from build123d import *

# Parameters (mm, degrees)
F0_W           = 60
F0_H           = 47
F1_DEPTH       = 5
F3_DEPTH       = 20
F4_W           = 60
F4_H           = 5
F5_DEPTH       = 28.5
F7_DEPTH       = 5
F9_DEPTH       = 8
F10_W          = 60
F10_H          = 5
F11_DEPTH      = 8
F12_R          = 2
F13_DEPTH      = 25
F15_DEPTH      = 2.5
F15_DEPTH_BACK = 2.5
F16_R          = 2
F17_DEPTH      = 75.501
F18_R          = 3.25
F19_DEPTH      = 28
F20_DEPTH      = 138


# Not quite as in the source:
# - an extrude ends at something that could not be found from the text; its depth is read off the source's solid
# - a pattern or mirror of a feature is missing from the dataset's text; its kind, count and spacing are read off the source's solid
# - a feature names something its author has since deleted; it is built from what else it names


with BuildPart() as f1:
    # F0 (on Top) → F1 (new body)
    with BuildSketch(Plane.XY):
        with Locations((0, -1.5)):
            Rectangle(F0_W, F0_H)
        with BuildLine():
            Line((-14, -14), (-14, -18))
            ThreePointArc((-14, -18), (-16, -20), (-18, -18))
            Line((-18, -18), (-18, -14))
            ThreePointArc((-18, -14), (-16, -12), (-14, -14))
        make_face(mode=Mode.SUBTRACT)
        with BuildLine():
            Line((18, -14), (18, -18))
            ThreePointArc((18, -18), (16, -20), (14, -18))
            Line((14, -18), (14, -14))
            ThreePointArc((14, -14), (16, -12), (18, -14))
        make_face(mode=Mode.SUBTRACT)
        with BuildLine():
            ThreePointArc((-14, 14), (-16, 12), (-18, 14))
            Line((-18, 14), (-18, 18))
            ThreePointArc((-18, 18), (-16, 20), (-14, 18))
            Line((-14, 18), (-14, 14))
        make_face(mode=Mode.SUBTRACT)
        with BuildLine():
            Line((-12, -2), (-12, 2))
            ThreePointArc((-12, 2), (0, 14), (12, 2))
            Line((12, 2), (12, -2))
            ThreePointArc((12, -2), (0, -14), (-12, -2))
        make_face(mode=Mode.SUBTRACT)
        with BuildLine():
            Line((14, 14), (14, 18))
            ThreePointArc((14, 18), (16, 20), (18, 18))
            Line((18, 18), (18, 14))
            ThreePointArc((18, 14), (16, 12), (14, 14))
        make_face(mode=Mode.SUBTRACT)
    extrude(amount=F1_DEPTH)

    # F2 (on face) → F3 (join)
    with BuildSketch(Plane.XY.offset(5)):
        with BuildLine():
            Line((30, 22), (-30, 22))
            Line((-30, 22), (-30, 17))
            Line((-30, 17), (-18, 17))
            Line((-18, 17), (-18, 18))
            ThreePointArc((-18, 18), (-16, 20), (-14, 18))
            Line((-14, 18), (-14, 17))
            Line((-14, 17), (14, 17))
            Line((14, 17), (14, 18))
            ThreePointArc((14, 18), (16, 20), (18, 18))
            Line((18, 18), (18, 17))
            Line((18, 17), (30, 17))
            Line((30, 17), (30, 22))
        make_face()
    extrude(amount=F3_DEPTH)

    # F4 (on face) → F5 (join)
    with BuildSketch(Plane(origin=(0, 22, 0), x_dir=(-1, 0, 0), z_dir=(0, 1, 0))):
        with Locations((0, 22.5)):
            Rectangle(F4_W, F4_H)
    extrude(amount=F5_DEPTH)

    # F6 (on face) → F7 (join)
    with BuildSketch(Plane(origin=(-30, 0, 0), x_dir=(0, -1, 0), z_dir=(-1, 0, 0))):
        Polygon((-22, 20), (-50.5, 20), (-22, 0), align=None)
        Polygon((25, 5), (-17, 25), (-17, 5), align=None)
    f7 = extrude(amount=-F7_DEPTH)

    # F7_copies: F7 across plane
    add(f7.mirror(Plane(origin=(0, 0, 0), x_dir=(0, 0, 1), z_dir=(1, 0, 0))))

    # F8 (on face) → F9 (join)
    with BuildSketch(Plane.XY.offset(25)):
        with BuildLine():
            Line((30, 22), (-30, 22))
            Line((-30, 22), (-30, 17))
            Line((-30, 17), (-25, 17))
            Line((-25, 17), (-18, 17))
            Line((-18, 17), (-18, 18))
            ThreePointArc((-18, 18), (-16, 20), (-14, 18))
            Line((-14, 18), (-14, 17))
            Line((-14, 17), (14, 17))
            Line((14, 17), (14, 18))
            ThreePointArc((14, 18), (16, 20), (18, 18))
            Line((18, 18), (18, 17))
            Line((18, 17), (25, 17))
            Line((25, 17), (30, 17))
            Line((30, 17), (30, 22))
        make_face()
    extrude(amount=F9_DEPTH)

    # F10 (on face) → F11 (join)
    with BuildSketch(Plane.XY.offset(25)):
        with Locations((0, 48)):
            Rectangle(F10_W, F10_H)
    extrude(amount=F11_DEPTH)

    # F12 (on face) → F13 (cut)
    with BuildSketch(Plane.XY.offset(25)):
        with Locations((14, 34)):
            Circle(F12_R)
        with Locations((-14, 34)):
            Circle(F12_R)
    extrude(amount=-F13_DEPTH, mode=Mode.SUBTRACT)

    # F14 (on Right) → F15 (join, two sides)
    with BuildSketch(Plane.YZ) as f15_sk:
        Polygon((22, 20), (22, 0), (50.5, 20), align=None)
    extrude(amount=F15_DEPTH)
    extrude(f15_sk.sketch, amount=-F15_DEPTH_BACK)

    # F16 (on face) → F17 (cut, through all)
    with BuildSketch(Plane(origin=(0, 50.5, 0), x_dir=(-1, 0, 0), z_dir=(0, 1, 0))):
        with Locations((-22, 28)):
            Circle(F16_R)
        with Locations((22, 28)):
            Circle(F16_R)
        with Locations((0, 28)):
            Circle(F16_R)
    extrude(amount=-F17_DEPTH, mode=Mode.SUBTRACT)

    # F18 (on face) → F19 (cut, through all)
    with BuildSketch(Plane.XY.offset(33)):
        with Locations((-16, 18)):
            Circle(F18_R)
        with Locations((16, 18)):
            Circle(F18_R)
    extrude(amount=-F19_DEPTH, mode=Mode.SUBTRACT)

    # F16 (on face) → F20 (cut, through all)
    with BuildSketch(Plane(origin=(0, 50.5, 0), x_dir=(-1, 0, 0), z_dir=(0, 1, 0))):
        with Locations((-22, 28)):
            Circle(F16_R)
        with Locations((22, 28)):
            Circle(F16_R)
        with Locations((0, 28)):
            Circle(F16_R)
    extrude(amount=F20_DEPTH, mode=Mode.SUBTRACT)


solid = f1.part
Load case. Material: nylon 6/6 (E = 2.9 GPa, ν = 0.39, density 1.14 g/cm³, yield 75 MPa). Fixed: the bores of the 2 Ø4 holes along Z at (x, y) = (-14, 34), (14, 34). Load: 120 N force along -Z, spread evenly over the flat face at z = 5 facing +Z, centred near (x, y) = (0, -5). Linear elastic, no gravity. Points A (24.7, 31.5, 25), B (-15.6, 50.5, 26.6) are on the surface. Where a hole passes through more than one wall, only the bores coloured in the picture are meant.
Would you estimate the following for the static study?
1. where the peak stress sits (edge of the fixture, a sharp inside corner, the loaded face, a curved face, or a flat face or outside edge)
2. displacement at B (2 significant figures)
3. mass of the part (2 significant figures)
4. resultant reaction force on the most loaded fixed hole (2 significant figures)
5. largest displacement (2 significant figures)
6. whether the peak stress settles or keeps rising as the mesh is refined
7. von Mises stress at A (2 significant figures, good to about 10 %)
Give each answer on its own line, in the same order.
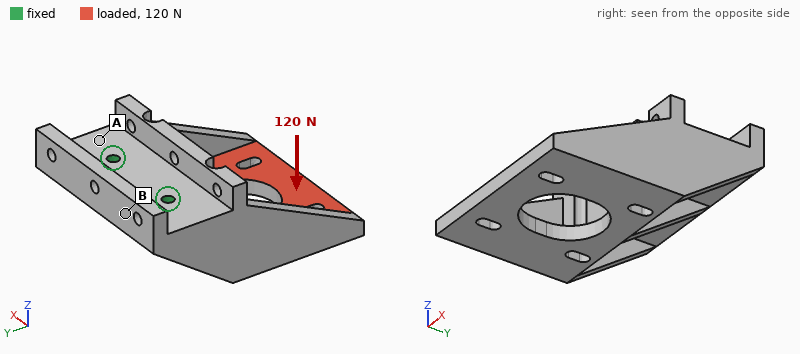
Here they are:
edge of the fixture
0.17 mm
42 g
61 N
1.1 mm
keeps rising
3.9 MPa
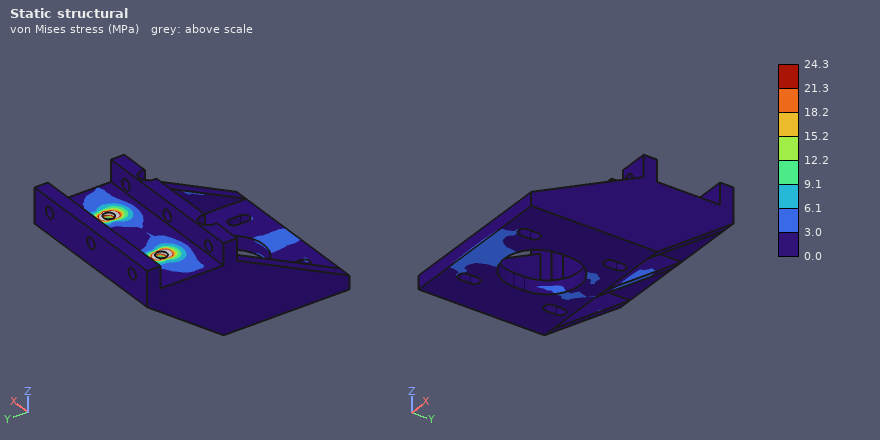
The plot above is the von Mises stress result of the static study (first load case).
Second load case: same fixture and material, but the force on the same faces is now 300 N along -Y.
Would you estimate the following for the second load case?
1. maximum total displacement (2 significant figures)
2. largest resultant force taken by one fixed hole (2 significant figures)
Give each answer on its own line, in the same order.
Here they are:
0.93 mm
150 N
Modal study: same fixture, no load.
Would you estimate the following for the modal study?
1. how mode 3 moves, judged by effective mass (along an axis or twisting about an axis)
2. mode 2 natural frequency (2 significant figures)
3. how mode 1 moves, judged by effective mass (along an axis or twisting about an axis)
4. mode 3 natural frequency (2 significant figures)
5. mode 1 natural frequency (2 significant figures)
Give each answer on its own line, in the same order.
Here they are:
along X
800 Hz
along Z
1300 Hz
510 Hz
